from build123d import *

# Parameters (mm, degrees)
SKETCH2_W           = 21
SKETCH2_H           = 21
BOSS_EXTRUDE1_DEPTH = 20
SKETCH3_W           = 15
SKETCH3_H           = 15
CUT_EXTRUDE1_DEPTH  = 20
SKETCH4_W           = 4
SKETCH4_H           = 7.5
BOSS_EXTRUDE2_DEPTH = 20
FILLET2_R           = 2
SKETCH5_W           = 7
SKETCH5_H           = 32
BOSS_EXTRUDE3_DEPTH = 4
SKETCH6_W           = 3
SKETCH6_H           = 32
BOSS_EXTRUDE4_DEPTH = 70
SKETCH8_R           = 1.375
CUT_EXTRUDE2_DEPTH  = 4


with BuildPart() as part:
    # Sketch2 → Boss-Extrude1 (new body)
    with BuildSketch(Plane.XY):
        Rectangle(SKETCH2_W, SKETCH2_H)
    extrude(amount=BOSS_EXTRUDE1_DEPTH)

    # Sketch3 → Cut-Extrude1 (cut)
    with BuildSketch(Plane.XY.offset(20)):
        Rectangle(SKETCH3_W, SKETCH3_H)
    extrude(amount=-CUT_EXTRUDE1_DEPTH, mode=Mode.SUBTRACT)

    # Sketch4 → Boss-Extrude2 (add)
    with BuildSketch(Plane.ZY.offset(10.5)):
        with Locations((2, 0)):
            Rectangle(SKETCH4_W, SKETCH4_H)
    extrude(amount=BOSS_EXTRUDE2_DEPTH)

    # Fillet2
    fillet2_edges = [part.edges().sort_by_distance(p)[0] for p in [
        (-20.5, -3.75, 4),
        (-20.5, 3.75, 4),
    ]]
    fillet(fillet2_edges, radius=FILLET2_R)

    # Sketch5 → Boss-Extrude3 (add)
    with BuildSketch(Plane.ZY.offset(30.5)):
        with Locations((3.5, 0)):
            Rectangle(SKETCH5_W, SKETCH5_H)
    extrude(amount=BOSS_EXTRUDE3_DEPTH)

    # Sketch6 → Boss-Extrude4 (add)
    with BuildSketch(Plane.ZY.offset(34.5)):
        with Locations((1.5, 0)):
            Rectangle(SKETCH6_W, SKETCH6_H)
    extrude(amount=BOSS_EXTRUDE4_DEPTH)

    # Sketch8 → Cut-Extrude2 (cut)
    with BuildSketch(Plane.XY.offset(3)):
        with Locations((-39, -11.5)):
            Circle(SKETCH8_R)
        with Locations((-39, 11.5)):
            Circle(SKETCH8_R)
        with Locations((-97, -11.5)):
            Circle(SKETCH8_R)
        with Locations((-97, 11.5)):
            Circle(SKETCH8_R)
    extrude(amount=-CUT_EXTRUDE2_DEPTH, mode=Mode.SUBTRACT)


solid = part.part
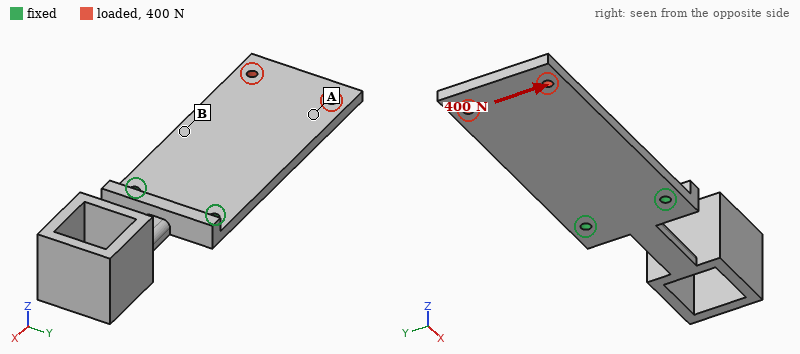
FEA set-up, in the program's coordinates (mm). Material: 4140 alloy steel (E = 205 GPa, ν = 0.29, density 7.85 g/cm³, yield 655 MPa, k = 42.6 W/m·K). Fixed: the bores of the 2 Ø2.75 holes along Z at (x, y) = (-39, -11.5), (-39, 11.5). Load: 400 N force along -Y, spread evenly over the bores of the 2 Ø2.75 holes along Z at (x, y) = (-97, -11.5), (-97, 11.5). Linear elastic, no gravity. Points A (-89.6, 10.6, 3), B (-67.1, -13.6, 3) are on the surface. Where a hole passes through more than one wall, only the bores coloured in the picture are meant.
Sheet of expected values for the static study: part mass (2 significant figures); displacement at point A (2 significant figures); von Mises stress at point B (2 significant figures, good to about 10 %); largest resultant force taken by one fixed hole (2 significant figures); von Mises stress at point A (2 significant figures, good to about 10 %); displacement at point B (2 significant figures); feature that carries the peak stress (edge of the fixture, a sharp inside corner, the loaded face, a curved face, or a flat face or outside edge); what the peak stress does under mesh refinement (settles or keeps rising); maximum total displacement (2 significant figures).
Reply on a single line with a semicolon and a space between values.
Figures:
98 g; 17 µm; 20 MPa; 990 N; 7.7 MPa; 8.1 µm; edge of the fixture; keeps rising; 24 µm
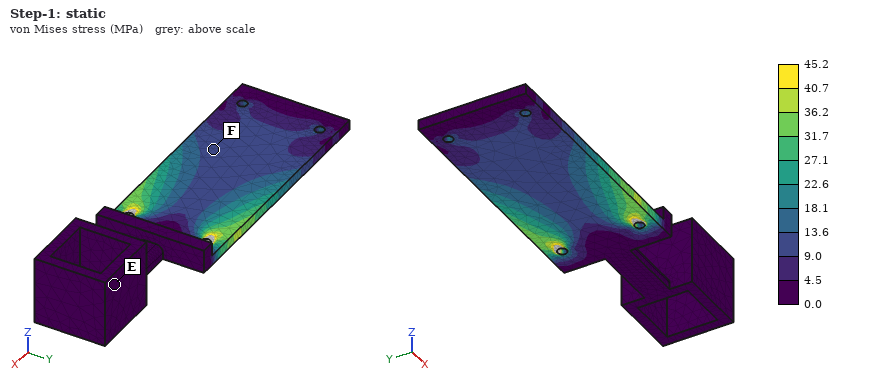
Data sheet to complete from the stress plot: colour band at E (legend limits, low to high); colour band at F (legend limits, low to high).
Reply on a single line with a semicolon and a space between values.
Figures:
0.0 to 4.5 MPa; 9.0 to 13.6 MPa
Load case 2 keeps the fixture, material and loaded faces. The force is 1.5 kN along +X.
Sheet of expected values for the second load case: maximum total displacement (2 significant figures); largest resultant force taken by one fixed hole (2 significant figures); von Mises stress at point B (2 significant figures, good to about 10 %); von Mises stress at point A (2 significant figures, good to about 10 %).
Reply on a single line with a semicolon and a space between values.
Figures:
5.6 µm; 750 N; 16 MPa; 20 MPa
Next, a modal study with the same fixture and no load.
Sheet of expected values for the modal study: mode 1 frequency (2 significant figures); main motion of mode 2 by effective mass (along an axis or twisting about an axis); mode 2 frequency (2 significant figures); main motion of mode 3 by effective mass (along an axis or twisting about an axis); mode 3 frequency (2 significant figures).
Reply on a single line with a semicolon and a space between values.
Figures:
510 Hz; along Z; 580 Hz; along Y; 930 Hz
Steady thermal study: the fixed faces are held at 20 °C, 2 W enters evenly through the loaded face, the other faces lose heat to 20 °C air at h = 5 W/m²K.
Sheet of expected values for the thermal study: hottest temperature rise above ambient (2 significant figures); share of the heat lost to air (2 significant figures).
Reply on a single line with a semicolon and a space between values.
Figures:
28 K; 18 %
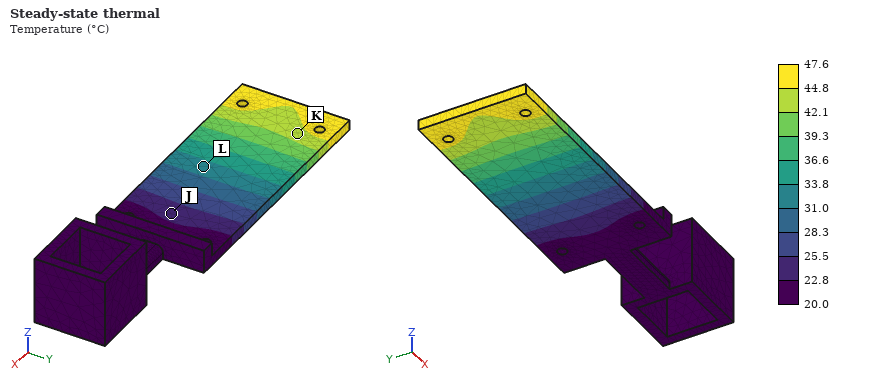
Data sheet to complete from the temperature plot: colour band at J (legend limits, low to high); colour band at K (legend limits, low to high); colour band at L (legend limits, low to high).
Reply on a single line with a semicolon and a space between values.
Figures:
22.8 to 25.5 °C; 42.1 to 44.8 °C; 31.0 to 33.8 °C
